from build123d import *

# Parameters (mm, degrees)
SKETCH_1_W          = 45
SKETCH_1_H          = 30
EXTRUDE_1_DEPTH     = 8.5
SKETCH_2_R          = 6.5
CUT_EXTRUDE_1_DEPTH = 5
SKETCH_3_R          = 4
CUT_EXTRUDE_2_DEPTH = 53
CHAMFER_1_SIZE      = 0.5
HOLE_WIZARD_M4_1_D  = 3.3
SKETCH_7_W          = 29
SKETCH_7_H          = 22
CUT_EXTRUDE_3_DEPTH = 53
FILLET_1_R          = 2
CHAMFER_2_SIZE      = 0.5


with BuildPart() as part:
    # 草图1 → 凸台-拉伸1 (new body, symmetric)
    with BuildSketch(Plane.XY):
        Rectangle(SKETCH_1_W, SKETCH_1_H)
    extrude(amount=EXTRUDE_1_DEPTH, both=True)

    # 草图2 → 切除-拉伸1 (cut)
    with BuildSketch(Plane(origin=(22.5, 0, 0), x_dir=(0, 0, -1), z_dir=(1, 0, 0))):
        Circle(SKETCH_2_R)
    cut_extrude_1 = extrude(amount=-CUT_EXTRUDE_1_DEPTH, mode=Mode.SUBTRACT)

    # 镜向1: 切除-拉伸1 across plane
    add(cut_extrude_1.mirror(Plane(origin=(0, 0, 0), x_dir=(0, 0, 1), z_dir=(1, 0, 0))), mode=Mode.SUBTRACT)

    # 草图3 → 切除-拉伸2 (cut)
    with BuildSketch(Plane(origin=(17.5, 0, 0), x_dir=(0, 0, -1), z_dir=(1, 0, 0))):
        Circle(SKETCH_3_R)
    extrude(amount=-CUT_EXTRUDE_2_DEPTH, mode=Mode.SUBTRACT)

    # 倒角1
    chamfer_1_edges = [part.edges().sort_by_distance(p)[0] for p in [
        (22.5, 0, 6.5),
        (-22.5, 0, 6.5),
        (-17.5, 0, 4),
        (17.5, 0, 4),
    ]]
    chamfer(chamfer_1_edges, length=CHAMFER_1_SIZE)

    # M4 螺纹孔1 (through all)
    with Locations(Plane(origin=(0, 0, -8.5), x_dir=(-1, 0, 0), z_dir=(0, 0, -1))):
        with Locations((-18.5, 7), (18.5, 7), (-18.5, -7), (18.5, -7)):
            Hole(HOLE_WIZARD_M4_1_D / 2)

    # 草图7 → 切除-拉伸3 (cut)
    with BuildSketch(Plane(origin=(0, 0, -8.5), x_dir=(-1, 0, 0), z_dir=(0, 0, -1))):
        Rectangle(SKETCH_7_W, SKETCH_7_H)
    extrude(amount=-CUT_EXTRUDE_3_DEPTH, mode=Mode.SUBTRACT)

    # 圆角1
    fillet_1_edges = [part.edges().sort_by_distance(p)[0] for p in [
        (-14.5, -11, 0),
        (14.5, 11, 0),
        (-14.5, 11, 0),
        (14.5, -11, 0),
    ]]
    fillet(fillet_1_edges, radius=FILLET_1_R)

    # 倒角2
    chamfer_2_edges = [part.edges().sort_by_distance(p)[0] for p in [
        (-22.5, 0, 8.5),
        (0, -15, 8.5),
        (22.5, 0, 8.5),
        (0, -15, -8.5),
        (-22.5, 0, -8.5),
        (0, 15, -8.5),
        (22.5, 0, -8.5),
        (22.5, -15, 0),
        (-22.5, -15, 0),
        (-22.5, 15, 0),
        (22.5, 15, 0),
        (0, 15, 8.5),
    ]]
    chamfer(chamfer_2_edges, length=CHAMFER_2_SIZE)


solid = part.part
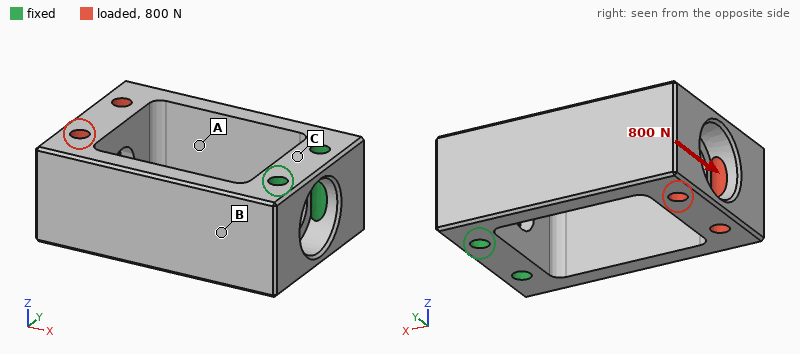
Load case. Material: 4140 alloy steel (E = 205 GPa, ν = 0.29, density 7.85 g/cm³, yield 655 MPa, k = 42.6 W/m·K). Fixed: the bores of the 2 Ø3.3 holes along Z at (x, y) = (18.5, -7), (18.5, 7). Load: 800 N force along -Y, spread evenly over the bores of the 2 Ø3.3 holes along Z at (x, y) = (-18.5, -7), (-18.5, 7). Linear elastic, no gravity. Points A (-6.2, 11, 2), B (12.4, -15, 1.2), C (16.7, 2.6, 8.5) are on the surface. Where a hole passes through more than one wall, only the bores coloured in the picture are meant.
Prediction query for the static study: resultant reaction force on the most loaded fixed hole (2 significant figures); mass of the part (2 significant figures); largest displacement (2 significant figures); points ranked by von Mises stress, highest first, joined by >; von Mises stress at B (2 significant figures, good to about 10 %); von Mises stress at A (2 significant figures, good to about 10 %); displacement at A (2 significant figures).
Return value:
910 N
78 g
76 µm
B > A > C
110 MPa
58 MPa
54 µm
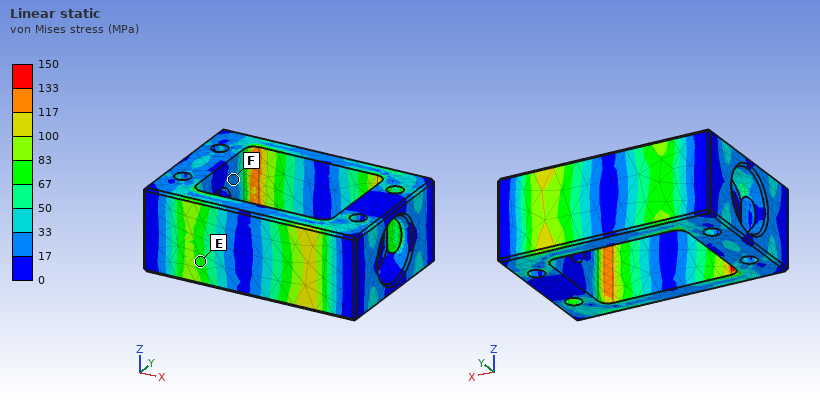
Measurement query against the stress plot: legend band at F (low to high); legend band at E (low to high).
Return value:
17 to 33 MPa
67 to 83 MPa
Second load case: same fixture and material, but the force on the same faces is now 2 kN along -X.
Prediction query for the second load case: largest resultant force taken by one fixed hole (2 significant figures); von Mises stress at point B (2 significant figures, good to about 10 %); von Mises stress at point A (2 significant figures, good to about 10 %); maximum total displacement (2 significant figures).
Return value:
1.0 kN
16 MPa
35 MPa
11 µm
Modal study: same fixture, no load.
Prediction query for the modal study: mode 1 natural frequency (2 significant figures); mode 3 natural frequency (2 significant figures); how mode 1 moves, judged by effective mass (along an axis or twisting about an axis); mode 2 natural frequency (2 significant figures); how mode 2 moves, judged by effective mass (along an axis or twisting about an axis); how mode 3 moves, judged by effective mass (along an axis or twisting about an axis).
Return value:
2800 Hz
7100 Hz
along Y
4600 Hz
along Z
twisting about X
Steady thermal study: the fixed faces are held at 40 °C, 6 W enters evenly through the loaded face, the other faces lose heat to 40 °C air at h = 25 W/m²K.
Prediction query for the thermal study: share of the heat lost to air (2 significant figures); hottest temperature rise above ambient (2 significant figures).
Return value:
32 %
29 K
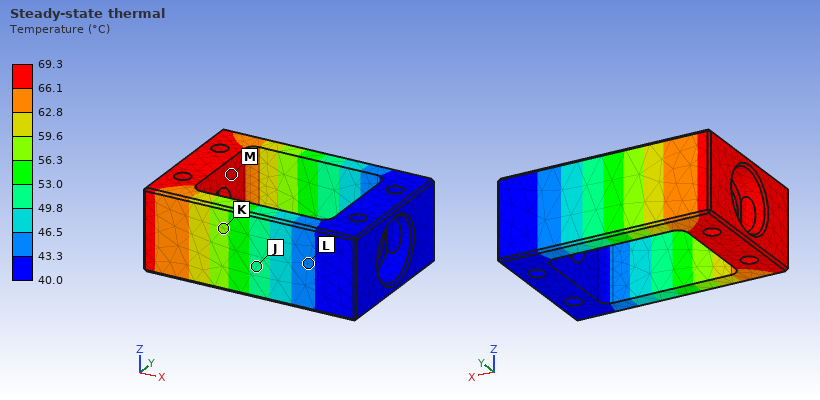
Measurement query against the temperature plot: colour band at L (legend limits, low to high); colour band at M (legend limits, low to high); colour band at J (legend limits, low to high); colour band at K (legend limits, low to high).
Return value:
43.3 to 46.5 °C
66.1 to 69.3 °C
49.8 to 53.0 °C
56.3 to 59.6 °C
